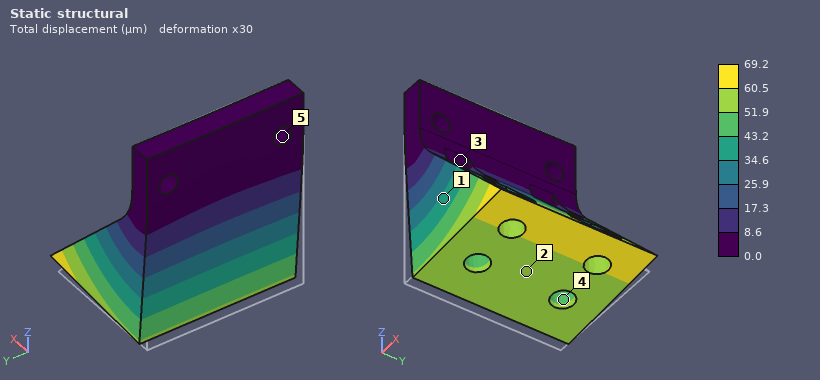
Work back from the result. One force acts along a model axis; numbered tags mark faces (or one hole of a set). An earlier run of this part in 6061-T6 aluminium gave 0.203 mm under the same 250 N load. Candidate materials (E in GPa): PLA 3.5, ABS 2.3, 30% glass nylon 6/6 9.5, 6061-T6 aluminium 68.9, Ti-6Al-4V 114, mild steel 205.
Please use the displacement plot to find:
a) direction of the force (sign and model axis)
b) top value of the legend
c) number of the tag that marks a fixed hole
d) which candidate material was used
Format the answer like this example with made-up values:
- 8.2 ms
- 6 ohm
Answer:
- +X
- 69.2 µm
- 5
- mild steel
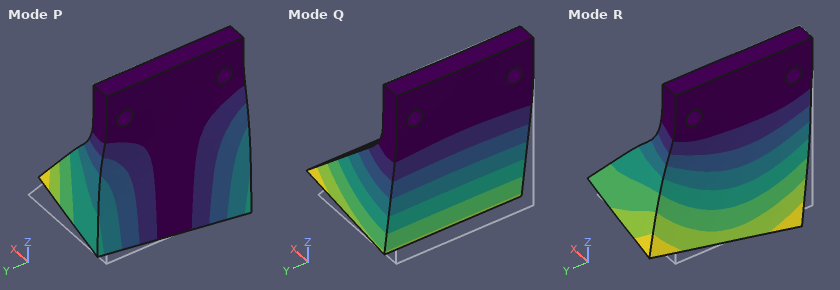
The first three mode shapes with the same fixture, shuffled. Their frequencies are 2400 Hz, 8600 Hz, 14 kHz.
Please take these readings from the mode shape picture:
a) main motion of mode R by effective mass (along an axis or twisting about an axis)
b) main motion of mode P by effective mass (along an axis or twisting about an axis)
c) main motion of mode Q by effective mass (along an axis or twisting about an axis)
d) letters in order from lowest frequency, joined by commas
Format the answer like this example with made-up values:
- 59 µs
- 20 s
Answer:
- along Y
- along Y
- along X
- Q, P, R
